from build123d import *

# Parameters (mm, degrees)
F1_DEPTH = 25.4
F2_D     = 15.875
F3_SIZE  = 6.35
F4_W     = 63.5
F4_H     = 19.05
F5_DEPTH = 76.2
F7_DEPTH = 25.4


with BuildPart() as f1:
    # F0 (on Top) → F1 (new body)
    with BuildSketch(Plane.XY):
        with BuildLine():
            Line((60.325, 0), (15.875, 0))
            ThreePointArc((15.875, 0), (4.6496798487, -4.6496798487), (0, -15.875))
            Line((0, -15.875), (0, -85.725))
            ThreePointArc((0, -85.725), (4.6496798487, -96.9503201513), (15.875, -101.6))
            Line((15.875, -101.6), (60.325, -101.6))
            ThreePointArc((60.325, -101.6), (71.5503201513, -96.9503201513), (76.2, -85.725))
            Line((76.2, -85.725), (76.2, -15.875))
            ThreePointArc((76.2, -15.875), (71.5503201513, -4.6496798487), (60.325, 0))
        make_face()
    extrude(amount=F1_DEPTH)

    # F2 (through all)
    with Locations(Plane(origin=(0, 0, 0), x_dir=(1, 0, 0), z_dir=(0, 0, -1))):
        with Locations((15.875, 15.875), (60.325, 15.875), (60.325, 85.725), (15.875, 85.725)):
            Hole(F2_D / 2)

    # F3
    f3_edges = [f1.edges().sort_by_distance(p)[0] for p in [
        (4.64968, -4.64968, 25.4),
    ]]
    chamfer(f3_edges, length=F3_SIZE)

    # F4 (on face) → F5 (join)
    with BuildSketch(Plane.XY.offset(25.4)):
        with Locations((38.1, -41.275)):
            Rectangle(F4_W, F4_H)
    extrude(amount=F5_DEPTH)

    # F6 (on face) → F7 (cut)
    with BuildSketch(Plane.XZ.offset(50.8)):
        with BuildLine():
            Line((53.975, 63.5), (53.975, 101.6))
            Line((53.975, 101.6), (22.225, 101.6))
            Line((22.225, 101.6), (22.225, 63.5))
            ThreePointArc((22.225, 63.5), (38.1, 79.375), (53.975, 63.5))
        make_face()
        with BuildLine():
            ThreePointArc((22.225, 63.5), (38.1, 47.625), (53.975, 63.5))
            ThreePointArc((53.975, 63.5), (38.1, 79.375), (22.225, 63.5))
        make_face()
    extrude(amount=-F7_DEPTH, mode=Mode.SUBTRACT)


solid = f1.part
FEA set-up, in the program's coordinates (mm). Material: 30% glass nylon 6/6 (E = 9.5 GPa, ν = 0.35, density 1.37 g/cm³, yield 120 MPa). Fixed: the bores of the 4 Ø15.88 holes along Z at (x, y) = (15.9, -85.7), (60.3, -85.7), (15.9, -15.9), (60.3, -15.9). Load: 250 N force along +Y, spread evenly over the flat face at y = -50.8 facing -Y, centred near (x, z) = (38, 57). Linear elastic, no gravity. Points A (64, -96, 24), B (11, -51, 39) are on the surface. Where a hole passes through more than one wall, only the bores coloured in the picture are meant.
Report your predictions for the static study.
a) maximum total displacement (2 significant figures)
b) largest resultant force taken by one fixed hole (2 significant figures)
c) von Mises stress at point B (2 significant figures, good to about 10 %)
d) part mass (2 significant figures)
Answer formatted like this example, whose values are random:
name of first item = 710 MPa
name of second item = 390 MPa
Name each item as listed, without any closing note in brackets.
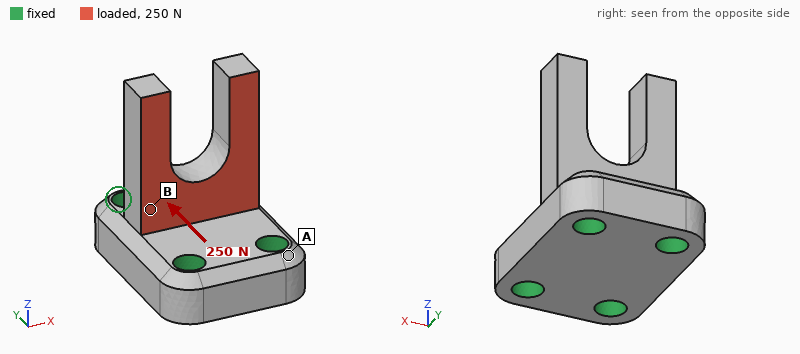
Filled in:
maximum total displacement = 55 µm
largest resultant force taken by one fixed hole = 130 N
von Mises stress at point B = 1.6 MPa
part mass = 310 g
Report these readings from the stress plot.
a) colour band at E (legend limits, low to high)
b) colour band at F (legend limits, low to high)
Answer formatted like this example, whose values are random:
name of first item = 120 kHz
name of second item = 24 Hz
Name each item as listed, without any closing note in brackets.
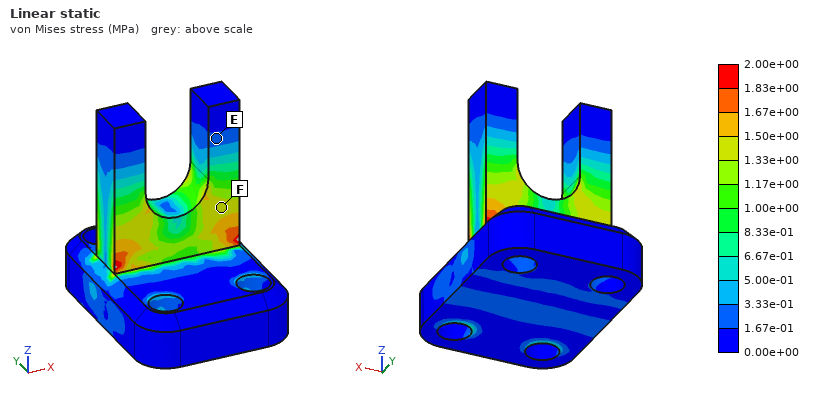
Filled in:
colour band at E = 1.67e-01 to 3.33e-01 MPa
colour band at F = 1.33e+00 to 1.50e+00 MPa
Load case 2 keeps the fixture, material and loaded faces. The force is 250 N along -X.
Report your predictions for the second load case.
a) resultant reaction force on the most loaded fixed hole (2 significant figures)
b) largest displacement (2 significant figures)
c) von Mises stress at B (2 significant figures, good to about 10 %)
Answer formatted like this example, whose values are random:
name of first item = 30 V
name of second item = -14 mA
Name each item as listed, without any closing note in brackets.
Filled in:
resultant reaction force on the most loaded fixed hole = 180 N
largest displacement = 37 µm
von Mises stress at B = 0.60 MPa
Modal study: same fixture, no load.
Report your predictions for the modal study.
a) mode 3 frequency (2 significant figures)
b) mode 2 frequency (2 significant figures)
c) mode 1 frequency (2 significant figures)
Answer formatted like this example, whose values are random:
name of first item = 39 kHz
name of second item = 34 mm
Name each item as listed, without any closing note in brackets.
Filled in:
mode 3 frequency = 1900 Hz
mode 2 frequency = 1600 Hz
mode 1 frequency = 1500 Hz
